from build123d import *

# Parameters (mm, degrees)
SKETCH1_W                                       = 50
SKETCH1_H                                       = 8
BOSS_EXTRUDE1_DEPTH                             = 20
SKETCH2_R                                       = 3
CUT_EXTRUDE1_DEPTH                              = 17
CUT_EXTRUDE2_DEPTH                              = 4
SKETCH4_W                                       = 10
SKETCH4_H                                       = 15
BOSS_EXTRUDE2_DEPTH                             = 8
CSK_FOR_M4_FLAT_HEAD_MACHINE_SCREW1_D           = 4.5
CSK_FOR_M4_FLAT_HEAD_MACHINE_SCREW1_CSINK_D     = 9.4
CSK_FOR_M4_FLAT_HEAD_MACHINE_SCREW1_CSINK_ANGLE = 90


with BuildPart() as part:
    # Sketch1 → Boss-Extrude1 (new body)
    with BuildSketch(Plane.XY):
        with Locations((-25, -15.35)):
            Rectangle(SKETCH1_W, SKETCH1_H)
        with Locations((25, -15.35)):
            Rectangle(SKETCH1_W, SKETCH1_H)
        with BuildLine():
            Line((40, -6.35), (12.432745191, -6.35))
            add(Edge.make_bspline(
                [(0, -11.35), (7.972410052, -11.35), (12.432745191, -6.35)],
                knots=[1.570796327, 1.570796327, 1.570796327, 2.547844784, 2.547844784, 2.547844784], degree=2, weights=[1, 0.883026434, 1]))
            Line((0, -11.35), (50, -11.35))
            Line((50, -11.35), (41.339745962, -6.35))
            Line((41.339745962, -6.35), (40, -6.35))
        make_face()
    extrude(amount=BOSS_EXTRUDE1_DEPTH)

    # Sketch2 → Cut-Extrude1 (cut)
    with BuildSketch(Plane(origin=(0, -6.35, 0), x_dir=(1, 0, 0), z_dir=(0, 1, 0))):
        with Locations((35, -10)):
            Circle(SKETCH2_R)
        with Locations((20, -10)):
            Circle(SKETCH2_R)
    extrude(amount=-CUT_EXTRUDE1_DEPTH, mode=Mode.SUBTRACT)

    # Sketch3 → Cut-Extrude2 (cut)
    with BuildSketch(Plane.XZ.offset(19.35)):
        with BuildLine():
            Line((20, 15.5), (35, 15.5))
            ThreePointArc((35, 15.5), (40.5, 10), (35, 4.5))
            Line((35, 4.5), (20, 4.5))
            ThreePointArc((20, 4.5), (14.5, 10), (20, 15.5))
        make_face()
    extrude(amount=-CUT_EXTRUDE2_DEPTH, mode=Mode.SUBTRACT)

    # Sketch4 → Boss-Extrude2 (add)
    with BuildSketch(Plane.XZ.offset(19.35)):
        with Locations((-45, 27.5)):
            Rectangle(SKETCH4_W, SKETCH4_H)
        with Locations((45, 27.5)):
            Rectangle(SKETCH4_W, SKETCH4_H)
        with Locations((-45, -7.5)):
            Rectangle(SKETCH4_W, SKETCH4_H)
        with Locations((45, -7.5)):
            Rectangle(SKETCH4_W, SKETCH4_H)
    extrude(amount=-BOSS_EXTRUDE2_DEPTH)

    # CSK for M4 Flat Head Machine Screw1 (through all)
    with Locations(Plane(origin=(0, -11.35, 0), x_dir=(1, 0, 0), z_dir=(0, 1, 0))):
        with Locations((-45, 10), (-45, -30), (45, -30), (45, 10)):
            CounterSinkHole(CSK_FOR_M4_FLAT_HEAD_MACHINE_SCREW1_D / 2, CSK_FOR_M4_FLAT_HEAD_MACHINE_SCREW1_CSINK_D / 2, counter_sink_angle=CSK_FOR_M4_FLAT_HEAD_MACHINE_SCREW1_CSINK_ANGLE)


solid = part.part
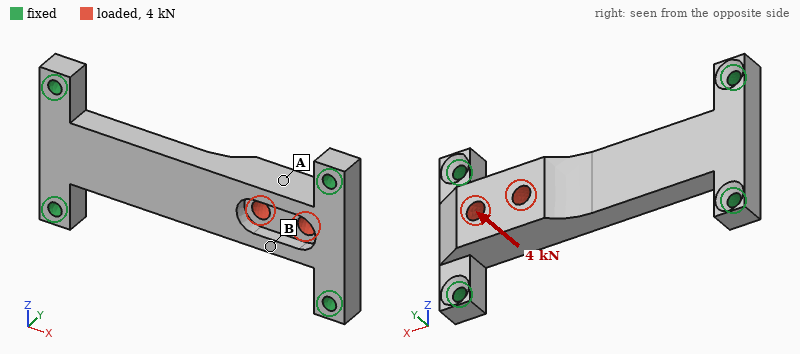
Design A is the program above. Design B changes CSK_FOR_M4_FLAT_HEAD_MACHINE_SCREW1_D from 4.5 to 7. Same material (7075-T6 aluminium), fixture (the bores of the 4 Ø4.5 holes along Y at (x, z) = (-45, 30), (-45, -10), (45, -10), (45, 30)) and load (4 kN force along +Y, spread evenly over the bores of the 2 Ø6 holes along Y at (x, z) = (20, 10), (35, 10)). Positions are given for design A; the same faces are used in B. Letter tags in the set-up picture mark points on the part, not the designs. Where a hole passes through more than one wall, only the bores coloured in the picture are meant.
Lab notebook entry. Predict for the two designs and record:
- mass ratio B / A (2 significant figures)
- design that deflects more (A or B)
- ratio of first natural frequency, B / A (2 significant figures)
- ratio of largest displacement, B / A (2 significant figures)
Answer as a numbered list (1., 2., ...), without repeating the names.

1. 0.97
2. A
3. 1.1
4. 0.87
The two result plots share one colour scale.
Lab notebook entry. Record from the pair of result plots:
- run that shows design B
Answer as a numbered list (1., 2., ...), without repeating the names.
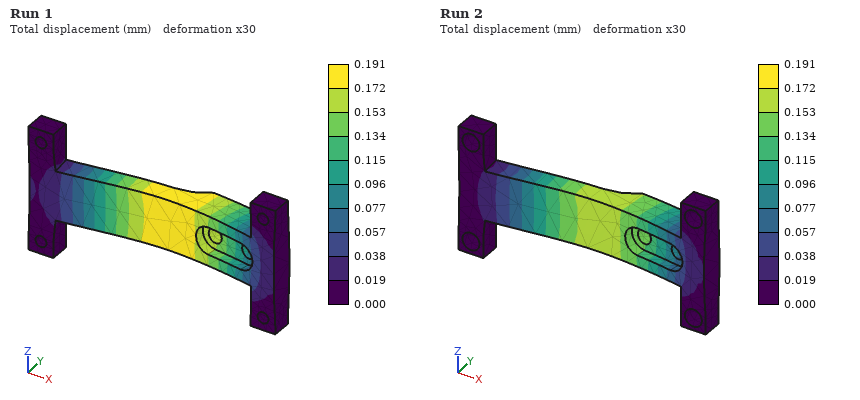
1. Run 2
